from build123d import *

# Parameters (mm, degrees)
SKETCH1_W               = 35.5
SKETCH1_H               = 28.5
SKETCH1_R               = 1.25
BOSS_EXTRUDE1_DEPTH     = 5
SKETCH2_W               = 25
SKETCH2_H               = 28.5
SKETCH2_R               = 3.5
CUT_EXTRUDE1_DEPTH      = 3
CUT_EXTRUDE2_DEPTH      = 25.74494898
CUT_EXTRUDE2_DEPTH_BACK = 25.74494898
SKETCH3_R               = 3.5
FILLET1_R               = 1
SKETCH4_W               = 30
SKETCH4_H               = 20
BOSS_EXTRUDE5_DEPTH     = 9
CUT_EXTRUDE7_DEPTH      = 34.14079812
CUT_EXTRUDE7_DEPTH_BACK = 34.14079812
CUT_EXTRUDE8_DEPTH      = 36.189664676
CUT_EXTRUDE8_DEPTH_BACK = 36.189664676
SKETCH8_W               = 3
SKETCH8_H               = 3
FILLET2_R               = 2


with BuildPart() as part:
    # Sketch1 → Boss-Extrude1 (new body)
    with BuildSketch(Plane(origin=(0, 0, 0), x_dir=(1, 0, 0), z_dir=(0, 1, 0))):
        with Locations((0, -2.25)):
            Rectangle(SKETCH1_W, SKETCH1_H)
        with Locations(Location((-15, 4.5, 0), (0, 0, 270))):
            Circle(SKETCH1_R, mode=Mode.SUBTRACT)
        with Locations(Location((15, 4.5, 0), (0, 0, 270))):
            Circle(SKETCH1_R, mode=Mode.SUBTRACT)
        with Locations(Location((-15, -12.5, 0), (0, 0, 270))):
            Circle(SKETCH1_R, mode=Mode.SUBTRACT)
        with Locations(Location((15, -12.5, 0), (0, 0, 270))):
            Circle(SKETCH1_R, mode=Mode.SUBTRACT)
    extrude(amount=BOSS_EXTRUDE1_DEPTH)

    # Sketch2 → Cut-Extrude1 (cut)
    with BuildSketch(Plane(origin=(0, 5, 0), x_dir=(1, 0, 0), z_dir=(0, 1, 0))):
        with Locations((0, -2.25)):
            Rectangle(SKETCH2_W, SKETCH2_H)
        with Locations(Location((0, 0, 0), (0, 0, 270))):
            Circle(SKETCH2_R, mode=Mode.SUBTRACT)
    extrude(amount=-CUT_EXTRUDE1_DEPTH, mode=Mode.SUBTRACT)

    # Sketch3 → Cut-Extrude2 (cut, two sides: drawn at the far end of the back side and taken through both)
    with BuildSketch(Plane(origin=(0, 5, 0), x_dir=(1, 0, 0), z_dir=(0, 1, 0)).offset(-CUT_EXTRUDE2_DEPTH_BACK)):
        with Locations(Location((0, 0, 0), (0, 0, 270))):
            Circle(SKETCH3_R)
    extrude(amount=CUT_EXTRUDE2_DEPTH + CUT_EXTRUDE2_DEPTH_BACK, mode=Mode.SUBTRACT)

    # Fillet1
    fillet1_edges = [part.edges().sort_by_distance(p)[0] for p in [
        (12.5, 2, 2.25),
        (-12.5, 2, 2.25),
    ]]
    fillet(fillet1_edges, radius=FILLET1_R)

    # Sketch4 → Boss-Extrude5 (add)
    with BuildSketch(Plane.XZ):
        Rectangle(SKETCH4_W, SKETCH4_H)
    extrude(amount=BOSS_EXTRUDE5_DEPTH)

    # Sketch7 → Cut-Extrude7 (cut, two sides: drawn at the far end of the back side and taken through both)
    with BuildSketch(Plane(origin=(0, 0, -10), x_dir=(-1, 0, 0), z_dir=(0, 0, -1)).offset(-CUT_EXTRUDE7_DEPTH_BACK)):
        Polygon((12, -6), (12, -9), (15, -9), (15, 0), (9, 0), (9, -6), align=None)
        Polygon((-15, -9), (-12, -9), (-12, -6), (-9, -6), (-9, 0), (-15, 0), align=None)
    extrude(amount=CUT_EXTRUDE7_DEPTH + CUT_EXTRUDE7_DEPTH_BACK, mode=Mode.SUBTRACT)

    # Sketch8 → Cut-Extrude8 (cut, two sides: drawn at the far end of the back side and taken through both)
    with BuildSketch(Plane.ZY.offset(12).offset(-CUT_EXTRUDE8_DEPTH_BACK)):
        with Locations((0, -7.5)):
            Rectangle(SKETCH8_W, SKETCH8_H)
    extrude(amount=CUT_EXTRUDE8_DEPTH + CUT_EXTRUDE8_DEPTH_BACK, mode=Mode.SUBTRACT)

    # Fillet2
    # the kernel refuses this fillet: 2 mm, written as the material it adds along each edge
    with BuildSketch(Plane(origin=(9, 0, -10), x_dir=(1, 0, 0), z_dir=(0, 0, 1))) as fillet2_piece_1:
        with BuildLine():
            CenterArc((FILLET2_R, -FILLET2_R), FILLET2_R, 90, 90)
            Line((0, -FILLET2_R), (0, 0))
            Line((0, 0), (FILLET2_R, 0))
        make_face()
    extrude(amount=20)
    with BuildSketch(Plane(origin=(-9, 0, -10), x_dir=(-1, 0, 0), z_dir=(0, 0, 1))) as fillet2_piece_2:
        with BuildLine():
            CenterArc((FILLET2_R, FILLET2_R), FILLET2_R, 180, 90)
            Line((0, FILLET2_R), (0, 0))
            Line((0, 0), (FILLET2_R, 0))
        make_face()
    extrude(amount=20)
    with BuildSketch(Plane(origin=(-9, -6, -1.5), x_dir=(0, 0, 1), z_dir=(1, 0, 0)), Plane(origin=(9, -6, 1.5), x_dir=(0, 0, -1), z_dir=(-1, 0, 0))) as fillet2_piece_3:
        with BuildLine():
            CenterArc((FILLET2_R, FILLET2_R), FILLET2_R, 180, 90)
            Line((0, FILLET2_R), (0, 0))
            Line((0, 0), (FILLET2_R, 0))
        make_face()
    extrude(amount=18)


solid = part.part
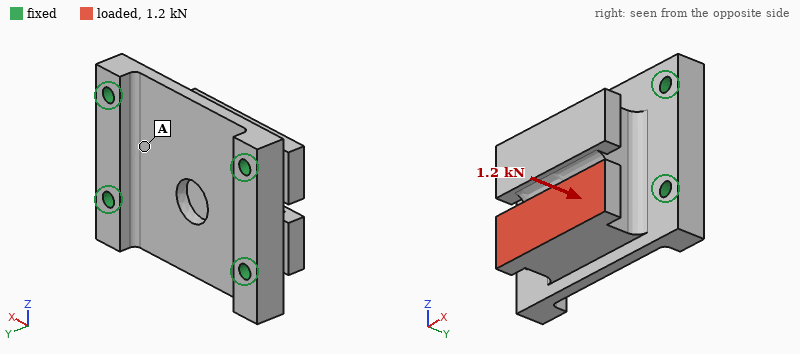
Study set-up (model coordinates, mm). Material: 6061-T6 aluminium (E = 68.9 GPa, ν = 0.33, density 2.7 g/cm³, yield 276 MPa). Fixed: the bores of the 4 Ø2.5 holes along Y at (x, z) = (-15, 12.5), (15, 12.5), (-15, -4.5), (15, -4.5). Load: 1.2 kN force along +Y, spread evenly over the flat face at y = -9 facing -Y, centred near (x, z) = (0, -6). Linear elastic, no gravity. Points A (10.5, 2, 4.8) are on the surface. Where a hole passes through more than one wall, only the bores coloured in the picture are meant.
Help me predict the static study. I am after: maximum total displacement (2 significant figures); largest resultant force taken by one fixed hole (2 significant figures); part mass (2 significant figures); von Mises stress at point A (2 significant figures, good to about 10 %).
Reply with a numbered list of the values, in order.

1. 25 µm
2. 740 N
3. 17 g
4. 15 MPa
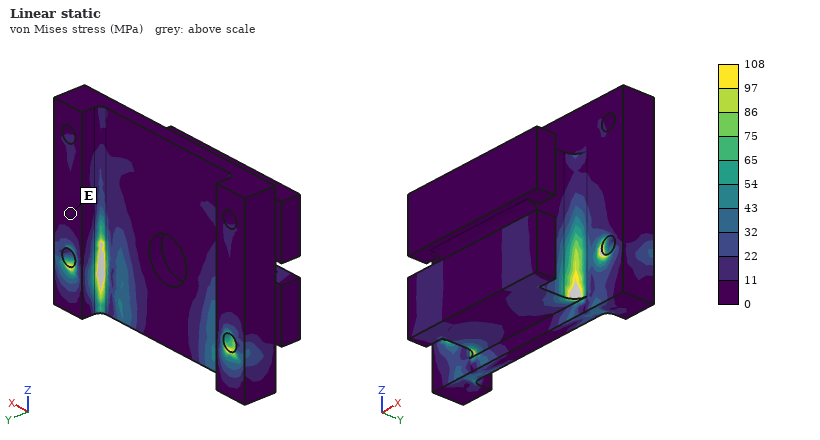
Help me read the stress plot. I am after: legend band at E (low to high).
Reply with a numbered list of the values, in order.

1. 0 to 11 MPa
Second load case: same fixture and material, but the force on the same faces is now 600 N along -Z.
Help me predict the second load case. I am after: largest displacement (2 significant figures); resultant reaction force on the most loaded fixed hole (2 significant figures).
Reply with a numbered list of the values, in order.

1. 16 µm
2. 300 N
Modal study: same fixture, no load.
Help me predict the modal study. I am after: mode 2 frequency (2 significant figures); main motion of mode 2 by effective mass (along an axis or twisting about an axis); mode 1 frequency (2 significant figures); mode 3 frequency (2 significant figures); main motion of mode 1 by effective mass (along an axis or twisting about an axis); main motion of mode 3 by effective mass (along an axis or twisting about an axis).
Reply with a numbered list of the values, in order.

1. 17 kHz
2. along Y
3. 14 kHz
4. 24 kHz
5. along Z
6. along X
